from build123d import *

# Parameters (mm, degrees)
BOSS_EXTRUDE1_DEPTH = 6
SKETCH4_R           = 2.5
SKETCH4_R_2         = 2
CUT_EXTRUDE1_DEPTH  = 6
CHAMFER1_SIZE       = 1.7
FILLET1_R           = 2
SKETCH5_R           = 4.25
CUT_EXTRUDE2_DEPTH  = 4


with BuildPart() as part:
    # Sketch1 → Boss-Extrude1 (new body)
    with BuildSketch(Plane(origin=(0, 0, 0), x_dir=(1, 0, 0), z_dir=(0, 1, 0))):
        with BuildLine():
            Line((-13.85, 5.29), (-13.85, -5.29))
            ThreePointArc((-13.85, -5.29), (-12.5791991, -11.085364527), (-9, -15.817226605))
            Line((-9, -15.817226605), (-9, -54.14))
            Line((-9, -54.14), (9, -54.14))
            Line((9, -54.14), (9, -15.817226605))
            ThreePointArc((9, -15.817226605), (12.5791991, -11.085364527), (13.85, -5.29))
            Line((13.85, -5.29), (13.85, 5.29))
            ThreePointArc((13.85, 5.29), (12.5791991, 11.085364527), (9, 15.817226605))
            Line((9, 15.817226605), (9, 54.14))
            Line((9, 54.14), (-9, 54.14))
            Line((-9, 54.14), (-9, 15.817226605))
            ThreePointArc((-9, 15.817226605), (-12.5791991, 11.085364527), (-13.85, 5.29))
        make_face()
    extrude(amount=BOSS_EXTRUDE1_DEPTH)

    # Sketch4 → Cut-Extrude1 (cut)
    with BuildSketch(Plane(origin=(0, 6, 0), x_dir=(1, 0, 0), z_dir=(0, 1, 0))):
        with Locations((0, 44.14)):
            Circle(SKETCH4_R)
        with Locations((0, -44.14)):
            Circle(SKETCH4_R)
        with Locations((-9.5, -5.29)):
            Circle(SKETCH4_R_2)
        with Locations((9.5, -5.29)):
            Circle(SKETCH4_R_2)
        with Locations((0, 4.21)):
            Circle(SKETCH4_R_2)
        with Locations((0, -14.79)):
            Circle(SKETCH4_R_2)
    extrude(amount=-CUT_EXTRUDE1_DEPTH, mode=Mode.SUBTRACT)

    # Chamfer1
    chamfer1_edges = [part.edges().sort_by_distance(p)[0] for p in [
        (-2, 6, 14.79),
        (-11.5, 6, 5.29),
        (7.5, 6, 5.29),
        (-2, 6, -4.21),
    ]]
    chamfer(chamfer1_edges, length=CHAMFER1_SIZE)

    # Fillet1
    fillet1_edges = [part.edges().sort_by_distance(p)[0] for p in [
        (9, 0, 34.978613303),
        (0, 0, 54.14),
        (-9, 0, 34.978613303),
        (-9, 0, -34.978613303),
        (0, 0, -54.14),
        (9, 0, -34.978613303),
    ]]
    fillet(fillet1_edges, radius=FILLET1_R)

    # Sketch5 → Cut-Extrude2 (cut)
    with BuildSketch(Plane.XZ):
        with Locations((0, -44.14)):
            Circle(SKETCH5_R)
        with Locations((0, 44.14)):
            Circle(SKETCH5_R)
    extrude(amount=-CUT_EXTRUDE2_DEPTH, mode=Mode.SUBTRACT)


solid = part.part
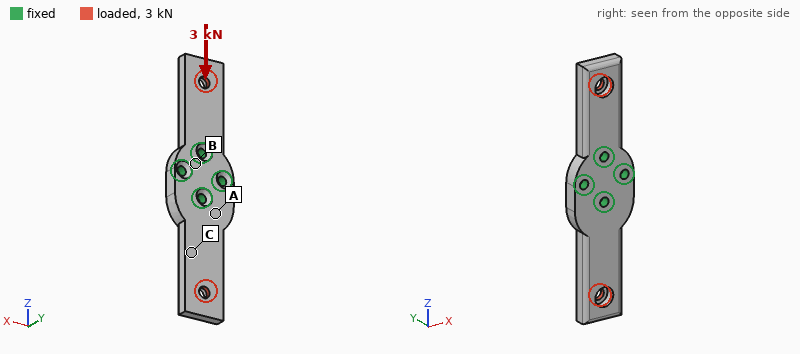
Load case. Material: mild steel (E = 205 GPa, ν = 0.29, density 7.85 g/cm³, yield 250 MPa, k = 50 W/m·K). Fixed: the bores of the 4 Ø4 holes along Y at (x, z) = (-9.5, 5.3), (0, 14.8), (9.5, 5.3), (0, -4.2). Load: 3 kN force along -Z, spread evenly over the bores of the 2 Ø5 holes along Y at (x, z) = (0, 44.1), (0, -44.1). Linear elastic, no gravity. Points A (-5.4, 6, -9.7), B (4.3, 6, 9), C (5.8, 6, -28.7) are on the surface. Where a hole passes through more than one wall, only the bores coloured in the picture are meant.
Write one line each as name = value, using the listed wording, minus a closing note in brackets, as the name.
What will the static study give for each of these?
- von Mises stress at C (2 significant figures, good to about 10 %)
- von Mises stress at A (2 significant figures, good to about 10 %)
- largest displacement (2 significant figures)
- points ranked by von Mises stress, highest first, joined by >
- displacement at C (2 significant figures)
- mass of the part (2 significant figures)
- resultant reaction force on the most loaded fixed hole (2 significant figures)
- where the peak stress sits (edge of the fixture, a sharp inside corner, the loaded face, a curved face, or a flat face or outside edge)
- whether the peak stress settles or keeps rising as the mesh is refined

von Mises stress at C = 42 MPa
von Mises stress at A = 32 MPa
largest displacement = 55 µm
points ranked by von Mises stress, highest first, joined by > = C > A > B
displacement at C = 15 µm
mass of the part = 95 g
resultant reaction force on the most loaded fixed hole = 980 N
where the peak stress sits = edge of the fixture
whether the peak stress settles or keeps rising as the mesh is refined = keeps rising
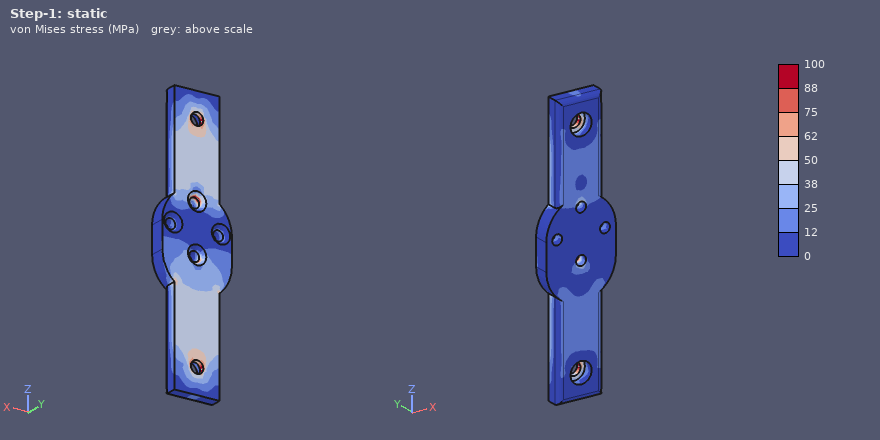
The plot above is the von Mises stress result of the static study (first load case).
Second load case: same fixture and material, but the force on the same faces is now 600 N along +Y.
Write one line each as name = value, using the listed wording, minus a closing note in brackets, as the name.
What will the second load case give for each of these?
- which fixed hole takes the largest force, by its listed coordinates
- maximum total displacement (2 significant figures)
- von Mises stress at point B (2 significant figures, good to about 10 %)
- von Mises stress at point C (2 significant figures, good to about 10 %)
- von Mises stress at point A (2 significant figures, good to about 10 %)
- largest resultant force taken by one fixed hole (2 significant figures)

which fixed hole takes the largest force, by its listed coordinates = (0, -4.2)
maximum total displacement = 0.13 mm
von Mises stress at point B = 12 MPa
von Mises stress at point C = 44 MPa
von Mises stress at point A = 71 MPa
largest resultant force taken by one fixed hole = 930 N
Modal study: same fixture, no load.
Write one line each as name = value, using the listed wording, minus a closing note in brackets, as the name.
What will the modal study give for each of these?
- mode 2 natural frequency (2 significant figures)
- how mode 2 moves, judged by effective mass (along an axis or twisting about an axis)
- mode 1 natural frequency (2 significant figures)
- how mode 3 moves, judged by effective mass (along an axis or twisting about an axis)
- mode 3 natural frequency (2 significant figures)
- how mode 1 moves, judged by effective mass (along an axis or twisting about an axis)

mode 2 natural frequency = 3200 Hz
how mode 2 moves, judged by effective mass = along Y
mode 1 natural frequency = 2100 Hz
how mode 3 moves, judged by effective mass = along X
mode 3 natural frequency = 6200 Hz
how mode 1 moves, judged by effective mass = along Y
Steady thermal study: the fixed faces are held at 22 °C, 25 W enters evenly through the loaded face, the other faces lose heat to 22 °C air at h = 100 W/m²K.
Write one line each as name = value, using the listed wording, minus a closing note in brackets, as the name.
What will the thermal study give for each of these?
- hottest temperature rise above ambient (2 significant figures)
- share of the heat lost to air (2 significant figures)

hottest temperature rise above ambient = 66 K
share of the heat lost to air = 52 %
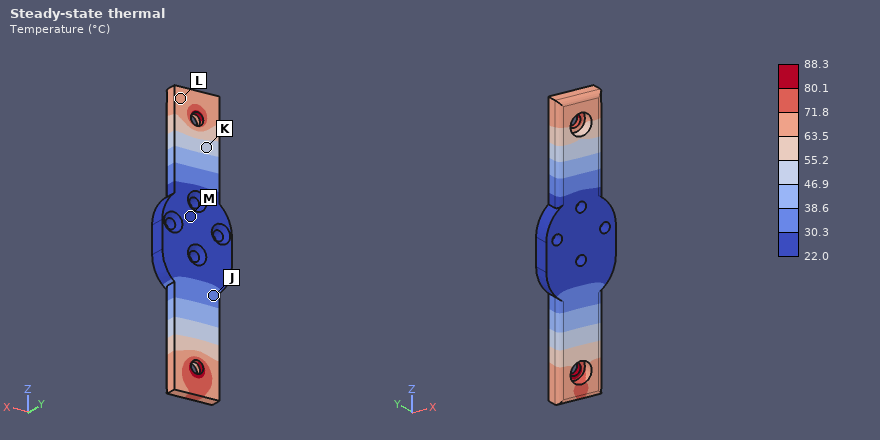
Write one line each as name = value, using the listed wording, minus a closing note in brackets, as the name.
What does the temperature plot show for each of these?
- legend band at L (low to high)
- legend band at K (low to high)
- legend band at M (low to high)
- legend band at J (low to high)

legend band at L = 63.5 to 71.8 °C
legend band at K = 46.9 to 55.2 °C
legend band at M = 22.0 to 30.3 °C
legend band at J = 30.3 to 38.6 °C
